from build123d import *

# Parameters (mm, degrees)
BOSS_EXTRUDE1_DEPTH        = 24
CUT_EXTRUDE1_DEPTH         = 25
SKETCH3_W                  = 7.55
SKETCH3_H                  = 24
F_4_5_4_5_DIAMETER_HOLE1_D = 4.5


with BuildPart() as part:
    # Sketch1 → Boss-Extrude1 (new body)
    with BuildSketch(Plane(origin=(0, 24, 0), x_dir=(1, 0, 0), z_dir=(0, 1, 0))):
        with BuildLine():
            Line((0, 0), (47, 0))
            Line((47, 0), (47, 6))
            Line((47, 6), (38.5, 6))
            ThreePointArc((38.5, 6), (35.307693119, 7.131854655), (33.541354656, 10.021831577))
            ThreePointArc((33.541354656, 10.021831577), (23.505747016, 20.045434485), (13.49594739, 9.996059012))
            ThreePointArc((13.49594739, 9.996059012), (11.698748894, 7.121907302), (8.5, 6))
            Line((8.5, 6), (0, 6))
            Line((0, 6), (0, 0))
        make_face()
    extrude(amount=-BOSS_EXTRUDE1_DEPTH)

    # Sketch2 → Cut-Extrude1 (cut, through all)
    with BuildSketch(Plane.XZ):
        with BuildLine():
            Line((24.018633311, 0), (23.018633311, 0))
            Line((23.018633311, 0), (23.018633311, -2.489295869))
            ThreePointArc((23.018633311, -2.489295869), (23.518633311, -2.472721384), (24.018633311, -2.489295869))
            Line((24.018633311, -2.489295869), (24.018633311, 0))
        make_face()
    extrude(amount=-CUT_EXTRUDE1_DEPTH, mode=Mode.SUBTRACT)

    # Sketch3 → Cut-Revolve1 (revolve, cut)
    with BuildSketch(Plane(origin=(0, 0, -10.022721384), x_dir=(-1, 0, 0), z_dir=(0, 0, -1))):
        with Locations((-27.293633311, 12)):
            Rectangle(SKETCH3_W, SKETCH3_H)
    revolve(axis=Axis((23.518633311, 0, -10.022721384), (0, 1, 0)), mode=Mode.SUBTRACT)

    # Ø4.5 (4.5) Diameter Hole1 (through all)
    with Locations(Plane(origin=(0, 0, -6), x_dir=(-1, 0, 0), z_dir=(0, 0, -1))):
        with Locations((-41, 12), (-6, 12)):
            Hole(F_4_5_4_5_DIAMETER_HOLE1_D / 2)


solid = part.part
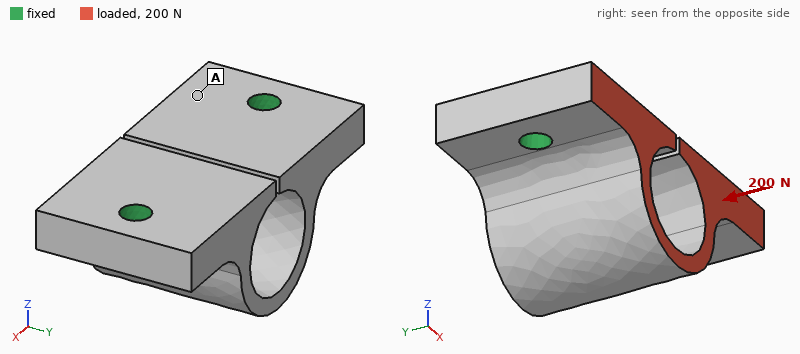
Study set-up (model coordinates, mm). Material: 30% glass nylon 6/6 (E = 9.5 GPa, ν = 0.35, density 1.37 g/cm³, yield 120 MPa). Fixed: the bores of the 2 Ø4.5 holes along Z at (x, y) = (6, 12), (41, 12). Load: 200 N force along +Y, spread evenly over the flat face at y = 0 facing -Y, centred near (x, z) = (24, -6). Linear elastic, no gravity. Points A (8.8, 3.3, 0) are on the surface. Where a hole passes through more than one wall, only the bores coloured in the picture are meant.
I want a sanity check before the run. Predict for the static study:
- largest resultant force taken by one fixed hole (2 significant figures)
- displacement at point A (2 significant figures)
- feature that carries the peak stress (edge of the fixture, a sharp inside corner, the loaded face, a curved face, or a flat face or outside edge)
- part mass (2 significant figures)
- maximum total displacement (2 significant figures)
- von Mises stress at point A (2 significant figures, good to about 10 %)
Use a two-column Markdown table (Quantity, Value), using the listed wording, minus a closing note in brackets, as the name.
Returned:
| Quantity | Value |
|---|---|
| largest resultant force taken by one fixed hole | 100 N |
| displacement at point A | 4.6 µm |
| feature that carries the peak stress | edge of the fixture |
| part mass | 11 g |
| maximum total displacement | 17 µm |
| von Mises stress at point A | 0.92 MPa |
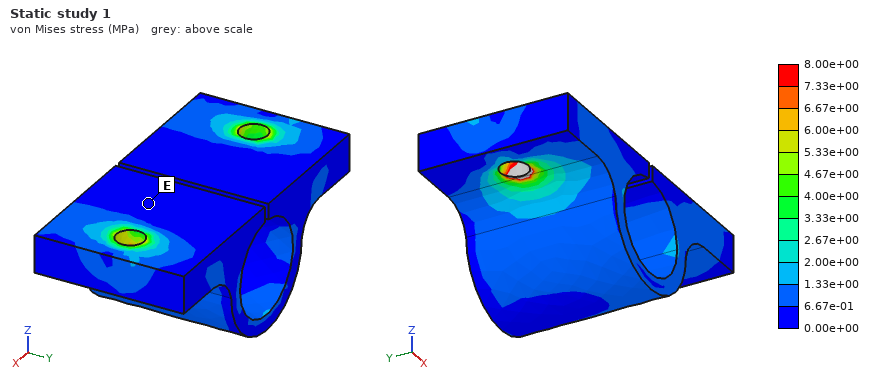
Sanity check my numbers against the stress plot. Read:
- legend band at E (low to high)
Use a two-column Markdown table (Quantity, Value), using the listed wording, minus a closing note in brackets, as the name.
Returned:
| Quantity | Value |
|---|---|
| legend band at E | 0.00e+00 to 6.67e-01 MPa |
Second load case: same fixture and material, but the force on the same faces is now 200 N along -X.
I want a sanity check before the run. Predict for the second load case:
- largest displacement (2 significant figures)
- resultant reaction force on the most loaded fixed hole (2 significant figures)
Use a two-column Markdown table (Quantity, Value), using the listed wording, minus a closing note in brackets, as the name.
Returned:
| Quantity | Value |
|---|---|
| largest displacement | 20 µm |
| resultant reaction force on the most loaded fixed hole | 100 N |
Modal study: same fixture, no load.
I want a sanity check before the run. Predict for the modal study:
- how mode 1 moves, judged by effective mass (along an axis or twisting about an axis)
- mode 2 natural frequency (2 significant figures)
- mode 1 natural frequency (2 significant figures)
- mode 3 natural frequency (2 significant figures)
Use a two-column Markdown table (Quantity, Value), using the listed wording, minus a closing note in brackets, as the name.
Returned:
| Quantity | Value |
|---|---|
| how mode 1 moves, judged by effective mass | along Y |
| mode 2 natural frequency | 7500 Hz |
| mode 1 natural frequency | 5900 Hz |
| mode 3 natural frequency | 8400 Hz |
